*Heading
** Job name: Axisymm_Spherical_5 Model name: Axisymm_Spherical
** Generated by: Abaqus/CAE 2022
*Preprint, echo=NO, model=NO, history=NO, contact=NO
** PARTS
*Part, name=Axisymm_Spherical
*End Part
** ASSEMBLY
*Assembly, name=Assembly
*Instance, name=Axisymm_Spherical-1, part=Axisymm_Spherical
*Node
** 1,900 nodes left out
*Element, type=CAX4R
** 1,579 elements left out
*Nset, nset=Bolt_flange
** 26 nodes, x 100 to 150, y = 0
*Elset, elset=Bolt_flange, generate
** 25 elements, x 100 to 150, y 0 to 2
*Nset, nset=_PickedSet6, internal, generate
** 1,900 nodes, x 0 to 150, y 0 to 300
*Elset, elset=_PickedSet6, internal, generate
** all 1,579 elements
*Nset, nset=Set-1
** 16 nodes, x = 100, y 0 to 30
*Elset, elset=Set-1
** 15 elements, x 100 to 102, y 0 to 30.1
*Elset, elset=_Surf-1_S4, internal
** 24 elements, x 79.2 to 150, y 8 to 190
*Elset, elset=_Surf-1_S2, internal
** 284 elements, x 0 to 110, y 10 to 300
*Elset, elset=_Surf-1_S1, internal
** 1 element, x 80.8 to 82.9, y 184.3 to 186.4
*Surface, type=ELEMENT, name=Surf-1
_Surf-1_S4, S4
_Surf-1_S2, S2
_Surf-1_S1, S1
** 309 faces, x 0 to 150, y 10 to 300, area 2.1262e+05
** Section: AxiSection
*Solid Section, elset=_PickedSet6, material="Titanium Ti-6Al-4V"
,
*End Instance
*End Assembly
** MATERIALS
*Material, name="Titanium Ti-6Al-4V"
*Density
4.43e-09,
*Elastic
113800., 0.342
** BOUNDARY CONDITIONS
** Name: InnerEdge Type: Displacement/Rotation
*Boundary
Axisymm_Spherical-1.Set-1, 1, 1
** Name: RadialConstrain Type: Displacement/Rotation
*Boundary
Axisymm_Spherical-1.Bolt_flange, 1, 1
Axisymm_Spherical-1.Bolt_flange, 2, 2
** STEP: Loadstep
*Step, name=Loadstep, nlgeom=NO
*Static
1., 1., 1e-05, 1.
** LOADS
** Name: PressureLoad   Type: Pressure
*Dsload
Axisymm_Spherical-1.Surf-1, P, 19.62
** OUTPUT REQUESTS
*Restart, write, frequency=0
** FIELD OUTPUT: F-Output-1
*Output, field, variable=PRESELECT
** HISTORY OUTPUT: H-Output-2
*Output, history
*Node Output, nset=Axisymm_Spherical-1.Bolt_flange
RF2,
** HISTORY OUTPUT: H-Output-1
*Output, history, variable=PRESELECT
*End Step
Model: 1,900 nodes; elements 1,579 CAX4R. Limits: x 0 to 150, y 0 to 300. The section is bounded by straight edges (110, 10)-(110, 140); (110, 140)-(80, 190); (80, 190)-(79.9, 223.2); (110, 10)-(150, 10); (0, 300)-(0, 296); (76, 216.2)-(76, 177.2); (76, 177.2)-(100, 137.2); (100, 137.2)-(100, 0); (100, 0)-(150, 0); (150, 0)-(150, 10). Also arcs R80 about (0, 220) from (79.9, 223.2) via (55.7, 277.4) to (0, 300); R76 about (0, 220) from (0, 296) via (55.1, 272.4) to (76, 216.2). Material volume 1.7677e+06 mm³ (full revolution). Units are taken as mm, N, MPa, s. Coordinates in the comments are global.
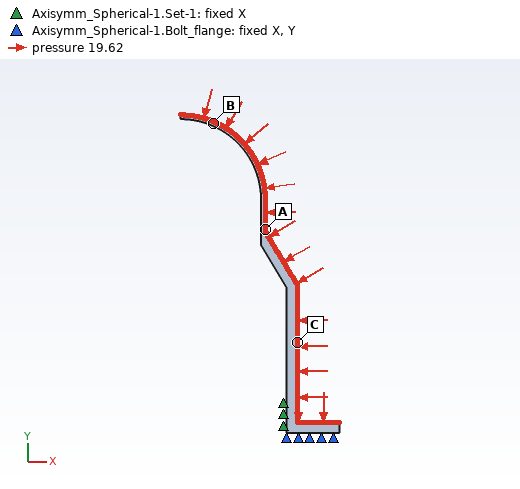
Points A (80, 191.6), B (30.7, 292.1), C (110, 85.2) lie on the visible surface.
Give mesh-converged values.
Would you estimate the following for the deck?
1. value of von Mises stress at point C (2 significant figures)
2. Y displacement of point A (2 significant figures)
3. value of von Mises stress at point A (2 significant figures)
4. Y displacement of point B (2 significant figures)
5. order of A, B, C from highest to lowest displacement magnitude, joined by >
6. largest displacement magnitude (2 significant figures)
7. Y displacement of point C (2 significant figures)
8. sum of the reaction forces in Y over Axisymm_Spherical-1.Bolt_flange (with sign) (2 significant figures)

190 MPa
-0.21 mm
510 MPa
-0.30 mm
A > B > C
0.37 mm
-0.050 mm
1.4e+06 N
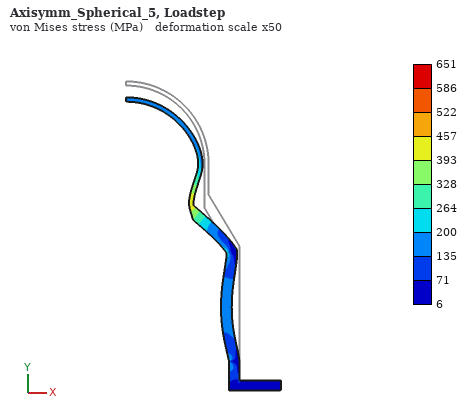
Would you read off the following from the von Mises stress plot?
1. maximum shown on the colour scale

651 MPa
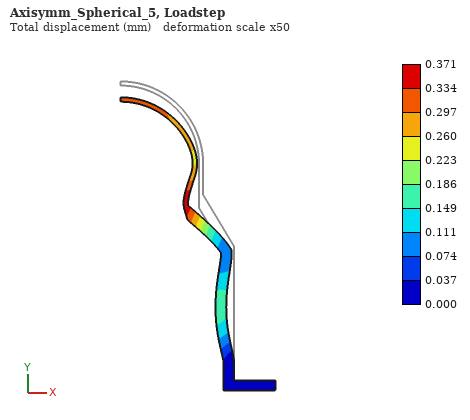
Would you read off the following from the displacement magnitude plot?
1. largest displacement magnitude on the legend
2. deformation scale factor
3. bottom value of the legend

0.371 mm
50
0.000 mm
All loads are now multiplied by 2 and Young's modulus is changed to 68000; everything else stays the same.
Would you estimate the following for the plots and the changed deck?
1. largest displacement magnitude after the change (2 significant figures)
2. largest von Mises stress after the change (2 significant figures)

1.2 mm
1300 MPa
